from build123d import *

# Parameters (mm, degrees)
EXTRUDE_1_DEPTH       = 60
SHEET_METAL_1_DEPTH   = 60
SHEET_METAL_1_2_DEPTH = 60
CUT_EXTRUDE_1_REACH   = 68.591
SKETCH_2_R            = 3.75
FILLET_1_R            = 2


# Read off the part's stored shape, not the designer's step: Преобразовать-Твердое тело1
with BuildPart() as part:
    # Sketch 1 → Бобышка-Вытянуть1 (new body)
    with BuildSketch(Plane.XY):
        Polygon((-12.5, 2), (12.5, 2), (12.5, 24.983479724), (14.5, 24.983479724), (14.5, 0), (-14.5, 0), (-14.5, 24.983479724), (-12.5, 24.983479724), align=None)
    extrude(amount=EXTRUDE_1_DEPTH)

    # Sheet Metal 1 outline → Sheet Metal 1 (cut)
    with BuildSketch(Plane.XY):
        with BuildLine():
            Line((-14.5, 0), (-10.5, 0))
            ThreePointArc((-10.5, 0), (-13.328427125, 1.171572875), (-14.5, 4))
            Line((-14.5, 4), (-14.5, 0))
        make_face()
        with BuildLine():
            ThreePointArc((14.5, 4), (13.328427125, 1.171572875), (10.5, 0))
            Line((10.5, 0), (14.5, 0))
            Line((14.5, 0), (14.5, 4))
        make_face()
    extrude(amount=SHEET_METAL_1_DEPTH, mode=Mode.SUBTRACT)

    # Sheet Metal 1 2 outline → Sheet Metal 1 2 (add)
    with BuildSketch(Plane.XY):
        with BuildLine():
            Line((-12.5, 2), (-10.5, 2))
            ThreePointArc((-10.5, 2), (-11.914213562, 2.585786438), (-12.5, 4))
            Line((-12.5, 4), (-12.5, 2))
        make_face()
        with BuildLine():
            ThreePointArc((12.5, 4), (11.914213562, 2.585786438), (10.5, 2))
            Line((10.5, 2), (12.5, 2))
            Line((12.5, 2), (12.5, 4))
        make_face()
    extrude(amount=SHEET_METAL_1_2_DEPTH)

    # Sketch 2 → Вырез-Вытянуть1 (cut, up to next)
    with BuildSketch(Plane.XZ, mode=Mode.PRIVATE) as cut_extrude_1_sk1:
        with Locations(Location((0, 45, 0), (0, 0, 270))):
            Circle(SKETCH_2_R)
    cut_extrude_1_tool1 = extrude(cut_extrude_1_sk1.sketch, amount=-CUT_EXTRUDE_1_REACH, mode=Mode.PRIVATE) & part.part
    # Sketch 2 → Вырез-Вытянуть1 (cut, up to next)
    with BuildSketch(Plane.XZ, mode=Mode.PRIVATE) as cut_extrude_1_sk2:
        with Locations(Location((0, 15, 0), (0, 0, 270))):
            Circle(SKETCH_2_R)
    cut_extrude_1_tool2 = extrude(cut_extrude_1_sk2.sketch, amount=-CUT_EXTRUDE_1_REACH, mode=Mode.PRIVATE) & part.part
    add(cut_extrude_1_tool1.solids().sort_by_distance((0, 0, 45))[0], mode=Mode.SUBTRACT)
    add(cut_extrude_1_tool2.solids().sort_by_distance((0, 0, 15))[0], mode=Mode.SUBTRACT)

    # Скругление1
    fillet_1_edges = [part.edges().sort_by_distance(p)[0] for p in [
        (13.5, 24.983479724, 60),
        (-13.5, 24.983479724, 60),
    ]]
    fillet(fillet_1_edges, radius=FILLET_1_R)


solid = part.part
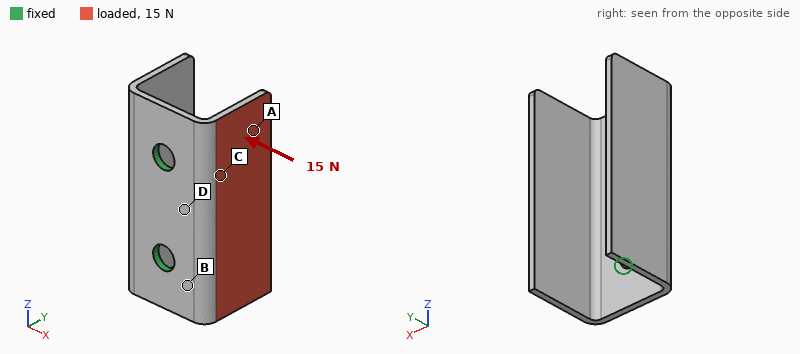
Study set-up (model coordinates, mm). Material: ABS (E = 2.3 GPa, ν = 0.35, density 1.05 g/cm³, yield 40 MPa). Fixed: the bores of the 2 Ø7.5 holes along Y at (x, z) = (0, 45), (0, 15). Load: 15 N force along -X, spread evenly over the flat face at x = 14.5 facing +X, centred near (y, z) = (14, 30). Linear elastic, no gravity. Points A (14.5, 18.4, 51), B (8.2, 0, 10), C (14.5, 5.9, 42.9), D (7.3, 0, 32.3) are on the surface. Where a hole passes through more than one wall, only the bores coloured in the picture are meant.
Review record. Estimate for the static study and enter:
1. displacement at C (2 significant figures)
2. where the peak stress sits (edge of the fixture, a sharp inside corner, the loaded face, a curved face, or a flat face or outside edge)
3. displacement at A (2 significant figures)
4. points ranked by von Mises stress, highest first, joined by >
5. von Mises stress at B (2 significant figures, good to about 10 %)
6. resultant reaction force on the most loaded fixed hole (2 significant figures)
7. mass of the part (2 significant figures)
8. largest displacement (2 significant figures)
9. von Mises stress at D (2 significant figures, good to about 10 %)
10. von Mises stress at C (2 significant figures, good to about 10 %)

0.21 mm
a flat face or outside edge
0.57 mm
B > D > C > A
4.6 MPa
7.5 N
8.9 g
0.80 mm
3.8 MPa
2.9 MPa
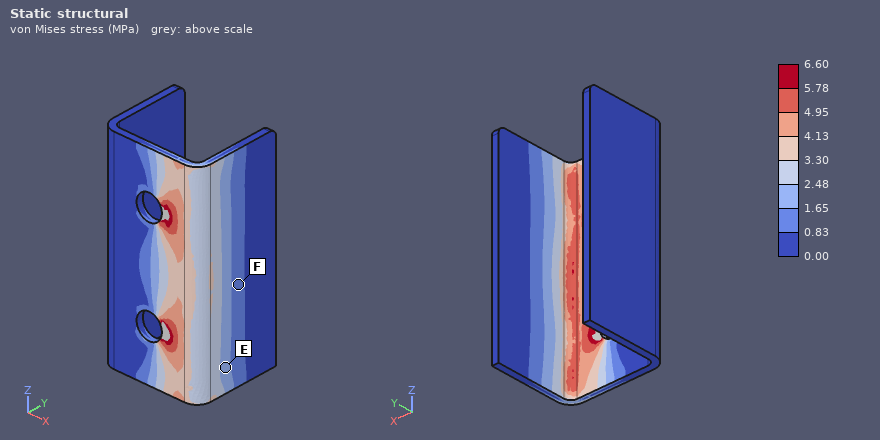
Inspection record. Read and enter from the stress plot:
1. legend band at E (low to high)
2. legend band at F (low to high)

1.65 to 2.48 MPa
0.83 to 1.65 MPa
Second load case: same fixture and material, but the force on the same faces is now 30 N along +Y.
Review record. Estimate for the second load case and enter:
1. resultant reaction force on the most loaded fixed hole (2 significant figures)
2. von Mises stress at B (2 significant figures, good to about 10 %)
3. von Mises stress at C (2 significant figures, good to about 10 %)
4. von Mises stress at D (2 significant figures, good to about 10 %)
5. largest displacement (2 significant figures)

15 N
4.8 MPa
0.78 MPa
3.5 MPa
0.67 mm
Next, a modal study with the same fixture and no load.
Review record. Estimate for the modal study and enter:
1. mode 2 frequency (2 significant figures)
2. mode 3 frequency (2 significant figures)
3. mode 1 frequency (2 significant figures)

500 Hz
750 Hz
500 Hz
